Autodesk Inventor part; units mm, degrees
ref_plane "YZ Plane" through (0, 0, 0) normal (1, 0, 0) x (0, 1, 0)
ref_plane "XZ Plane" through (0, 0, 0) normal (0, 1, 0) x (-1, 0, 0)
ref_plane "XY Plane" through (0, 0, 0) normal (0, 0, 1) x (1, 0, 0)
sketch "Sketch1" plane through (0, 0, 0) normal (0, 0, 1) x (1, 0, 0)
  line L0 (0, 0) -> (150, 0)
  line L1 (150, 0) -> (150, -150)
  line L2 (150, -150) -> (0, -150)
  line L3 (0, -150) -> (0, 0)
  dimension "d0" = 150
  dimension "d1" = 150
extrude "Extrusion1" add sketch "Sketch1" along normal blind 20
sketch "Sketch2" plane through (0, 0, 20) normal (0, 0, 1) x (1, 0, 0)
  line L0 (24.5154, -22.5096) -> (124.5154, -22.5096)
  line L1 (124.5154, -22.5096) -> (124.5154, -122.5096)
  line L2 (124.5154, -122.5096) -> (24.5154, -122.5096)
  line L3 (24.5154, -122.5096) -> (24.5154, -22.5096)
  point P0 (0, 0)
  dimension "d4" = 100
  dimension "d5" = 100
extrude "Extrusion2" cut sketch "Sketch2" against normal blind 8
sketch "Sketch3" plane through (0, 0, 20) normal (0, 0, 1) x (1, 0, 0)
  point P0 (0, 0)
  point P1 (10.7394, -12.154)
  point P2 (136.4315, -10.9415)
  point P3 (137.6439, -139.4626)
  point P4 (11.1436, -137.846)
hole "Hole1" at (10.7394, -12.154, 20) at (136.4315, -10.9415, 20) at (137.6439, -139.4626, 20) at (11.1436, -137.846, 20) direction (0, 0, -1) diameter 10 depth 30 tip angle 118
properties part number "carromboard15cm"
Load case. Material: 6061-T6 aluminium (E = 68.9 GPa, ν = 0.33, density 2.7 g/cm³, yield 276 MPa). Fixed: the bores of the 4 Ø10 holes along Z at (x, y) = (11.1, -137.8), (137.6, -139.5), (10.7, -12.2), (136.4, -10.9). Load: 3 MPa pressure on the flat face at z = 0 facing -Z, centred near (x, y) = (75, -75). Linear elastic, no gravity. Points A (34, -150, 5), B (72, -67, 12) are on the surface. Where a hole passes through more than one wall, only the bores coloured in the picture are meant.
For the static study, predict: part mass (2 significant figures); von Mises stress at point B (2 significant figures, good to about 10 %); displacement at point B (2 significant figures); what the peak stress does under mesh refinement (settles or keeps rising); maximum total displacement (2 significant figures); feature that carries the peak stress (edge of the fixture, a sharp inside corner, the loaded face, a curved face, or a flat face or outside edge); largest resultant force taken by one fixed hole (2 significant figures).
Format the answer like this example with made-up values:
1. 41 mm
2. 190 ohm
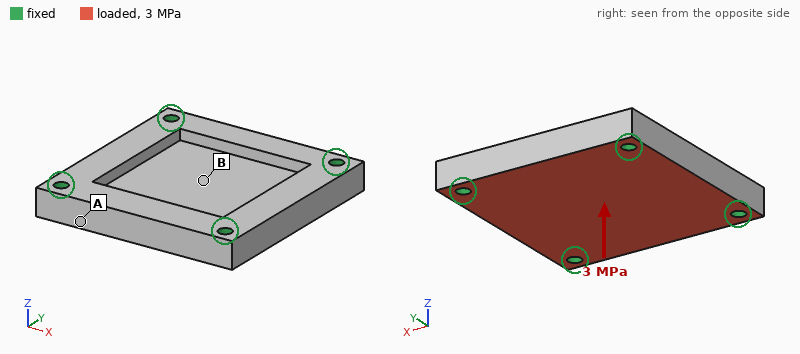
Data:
1. 980 g
2. 59 MPa
3. 0.24 mm
4. keeps rising
5. 0.25 mm
6. edge of the fixture
7. 18 kN
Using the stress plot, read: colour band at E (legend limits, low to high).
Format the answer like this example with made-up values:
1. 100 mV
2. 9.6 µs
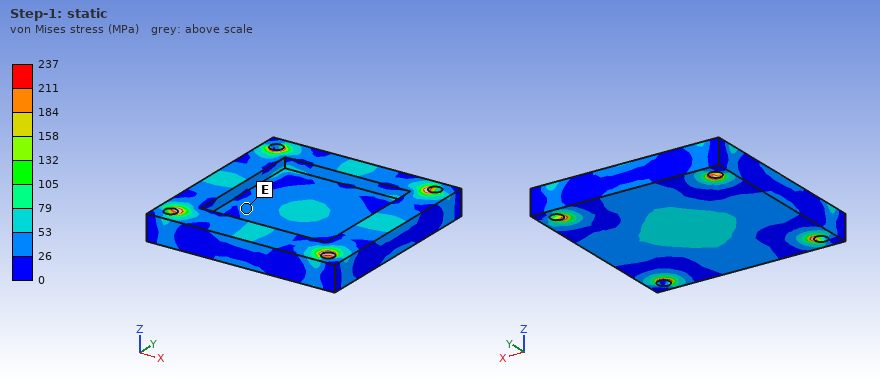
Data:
1. 26 to 53 MPa
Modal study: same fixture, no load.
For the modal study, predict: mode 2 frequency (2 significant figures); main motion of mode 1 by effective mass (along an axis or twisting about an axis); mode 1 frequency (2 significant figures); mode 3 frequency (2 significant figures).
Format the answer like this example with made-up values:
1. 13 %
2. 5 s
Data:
1. 5700 Hz
2. along Z
3. 3700 Hz
4. 5800 Hz
